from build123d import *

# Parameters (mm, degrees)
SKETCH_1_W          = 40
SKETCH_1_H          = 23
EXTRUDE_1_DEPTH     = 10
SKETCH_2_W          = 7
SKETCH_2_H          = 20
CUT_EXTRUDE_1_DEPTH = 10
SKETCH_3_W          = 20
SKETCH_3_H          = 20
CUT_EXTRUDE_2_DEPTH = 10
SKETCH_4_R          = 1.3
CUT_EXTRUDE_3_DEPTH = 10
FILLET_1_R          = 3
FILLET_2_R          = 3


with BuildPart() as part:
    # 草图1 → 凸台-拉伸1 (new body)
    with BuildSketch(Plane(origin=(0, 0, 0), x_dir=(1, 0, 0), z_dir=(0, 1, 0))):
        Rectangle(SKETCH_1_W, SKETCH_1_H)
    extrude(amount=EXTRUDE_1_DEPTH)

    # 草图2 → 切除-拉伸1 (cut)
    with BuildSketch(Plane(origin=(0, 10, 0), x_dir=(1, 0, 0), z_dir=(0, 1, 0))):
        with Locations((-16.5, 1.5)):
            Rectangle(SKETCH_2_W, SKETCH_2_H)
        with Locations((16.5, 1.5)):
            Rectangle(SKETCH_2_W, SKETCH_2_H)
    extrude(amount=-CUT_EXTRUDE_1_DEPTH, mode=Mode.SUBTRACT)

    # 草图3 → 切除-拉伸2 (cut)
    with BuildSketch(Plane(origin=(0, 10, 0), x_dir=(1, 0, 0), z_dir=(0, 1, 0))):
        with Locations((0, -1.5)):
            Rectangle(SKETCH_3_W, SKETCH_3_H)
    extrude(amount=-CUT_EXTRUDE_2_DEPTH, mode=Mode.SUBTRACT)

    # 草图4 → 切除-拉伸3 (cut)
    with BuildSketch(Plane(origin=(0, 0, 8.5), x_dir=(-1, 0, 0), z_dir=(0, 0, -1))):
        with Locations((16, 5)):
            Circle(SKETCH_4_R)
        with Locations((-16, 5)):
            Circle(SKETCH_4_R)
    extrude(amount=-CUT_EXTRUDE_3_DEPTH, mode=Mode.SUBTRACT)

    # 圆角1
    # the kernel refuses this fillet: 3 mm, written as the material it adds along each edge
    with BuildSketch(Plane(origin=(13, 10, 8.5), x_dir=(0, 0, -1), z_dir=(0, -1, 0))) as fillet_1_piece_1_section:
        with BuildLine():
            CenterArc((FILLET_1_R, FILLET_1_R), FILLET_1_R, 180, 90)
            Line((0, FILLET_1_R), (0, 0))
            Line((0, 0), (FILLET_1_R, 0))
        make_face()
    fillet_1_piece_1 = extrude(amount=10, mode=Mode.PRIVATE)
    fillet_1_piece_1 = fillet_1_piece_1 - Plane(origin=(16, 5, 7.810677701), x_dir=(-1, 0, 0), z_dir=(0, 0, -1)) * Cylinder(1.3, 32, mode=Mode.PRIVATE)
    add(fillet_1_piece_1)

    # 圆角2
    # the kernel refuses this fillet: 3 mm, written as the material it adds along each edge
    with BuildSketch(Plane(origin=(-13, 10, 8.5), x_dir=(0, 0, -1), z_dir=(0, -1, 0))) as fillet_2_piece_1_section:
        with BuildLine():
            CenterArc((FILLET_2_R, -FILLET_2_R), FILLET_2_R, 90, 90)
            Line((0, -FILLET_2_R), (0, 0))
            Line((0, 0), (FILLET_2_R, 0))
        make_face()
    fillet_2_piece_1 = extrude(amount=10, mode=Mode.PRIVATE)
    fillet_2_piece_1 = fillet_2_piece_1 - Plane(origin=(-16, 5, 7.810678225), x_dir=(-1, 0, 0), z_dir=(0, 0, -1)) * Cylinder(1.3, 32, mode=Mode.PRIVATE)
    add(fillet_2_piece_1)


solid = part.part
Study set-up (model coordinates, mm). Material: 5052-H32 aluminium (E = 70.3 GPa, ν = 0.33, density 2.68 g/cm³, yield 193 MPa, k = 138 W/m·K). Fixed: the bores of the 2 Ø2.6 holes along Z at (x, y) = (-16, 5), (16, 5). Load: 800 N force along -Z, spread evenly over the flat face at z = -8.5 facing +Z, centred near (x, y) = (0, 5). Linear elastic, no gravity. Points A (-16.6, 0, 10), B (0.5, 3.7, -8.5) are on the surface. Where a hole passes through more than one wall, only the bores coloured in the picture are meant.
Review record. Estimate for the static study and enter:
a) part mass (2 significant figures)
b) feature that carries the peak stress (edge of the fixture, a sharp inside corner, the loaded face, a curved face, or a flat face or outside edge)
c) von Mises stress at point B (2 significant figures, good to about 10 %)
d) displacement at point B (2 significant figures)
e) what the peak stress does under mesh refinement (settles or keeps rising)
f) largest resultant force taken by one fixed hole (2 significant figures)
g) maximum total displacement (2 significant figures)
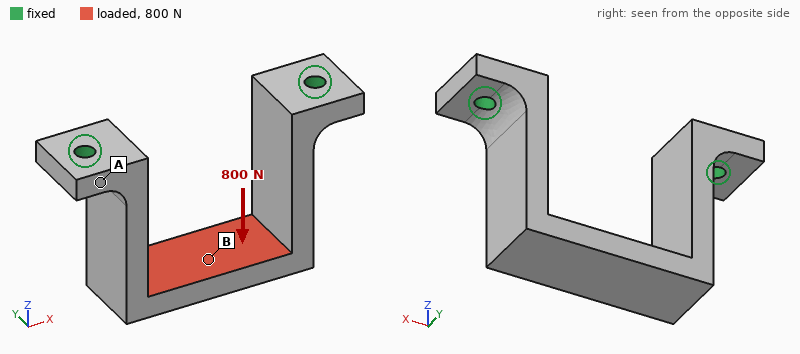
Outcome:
6.4 g
edge of the fixture
72 MPa
40 µm
keeps rising
420 N
43 µm
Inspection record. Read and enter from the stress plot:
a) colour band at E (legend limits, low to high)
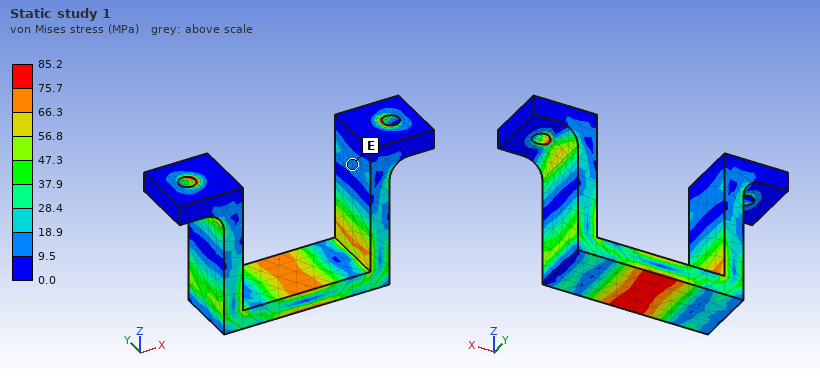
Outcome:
9.5 to 18.9 MPa
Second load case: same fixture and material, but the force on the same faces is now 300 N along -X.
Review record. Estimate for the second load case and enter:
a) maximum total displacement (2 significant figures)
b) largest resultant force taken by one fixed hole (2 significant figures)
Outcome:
88 µm
180 N
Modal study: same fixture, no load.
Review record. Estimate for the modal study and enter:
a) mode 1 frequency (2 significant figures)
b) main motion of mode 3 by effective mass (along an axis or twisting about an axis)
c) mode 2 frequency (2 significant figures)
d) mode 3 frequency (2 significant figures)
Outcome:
5400 Hz
twisting about Z
5500 Hz
8900 Hz
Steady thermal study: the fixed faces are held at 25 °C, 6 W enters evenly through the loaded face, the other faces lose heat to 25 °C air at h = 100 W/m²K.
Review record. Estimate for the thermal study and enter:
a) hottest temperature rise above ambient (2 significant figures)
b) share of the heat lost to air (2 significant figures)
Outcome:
16 K
22 %
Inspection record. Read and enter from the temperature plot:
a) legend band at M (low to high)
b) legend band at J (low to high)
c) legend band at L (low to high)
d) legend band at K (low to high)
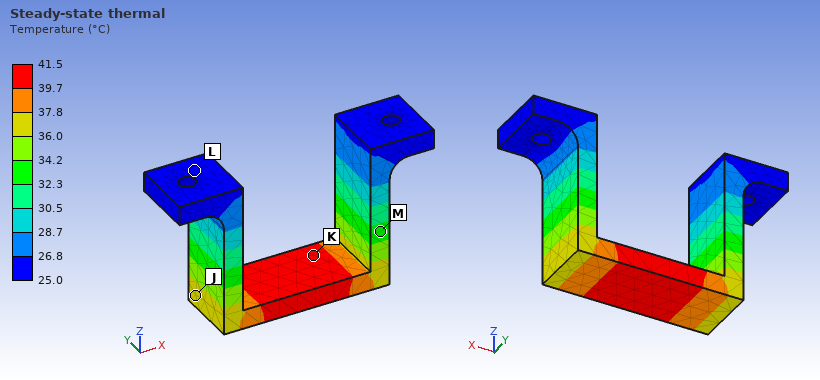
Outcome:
32.3 to 34.2 °C
36.0 to 37.8 °C
25.0 to 26.8 °C
39.7 to 41.5 °C
